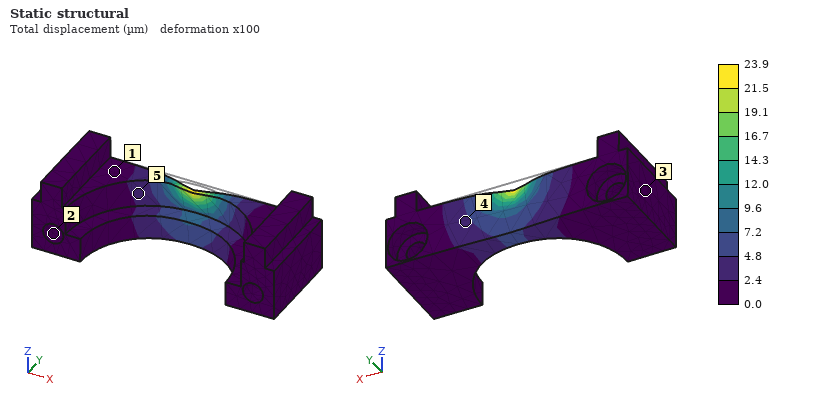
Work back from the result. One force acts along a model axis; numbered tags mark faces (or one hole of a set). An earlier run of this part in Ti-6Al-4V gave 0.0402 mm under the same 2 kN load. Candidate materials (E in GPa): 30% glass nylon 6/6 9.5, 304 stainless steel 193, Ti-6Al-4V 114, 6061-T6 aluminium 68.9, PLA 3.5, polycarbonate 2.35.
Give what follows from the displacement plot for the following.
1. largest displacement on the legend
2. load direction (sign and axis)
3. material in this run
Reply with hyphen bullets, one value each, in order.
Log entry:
- 23.9 µm
- -Y
- 304 stainless steel
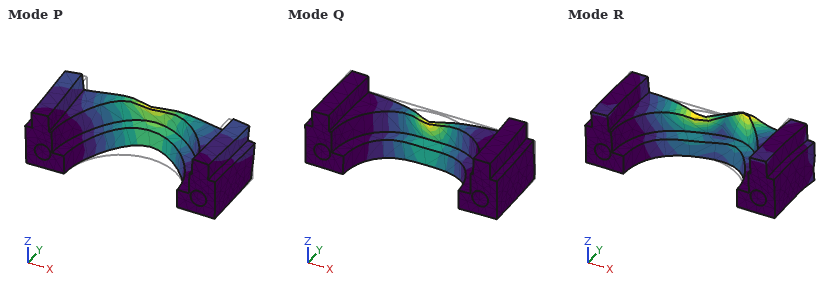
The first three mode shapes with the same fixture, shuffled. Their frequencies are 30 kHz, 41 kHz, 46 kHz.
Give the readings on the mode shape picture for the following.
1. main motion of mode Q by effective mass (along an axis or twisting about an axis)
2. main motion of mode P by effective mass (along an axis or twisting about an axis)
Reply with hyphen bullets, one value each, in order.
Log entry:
- along Y
- along Z
